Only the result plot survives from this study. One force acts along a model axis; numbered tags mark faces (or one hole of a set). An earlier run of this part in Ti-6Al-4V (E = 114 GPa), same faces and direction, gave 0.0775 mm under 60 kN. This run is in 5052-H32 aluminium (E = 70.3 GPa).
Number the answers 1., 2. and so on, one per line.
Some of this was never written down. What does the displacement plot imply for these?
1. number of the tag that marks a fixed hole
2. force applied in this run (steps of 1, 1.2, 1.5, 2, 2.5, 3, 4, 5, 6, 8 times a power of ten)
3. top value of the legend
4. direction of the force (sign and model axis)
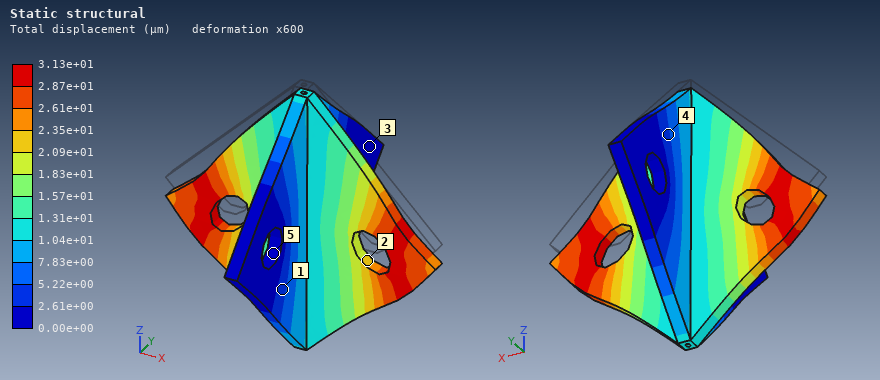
1. 5
2. 15 kN
3. 3.13e+01 µm
4. -Z
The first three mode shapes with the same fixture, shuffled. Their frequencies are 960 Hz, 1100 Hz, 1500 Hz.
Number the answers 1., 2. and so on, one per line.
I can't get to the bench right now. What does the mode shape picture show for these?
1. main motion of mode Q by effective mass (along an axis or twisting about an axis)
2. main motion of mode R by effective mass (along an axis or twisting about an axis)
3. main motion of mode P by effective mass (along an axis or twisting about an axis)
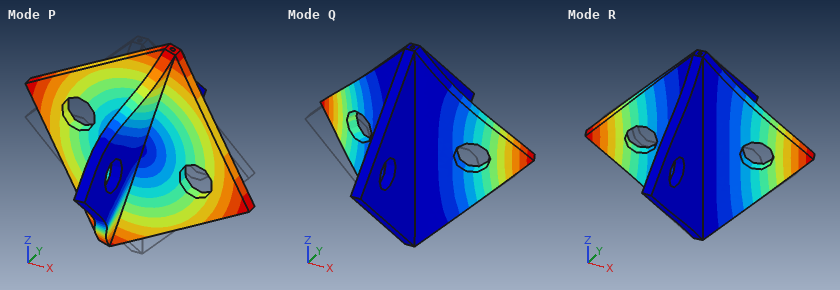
1. along Y
2. twisting about Z
3. twisting about Y
